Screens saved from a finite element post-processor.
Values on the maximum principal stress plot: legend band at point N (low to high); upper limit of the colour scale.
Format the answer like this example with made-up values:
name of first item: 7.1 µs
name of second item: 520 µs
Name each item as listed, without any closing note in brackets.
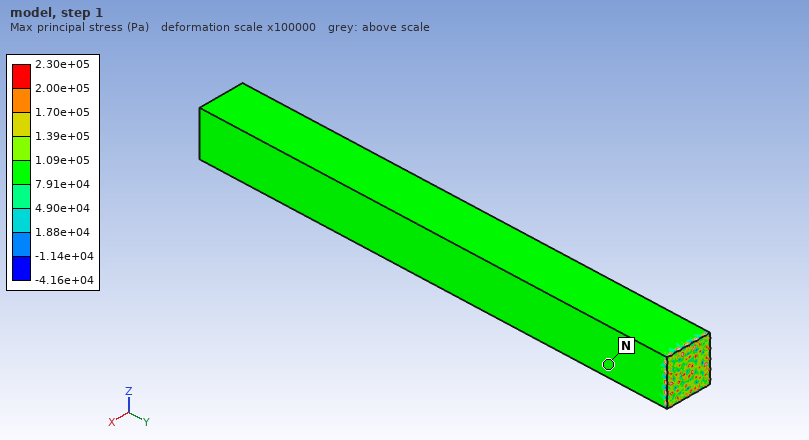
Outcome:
legend band at point N: 7.91e+04 to 1.09e+05 Pa
upper limit of the colour scale: 2.30e+05 Pa
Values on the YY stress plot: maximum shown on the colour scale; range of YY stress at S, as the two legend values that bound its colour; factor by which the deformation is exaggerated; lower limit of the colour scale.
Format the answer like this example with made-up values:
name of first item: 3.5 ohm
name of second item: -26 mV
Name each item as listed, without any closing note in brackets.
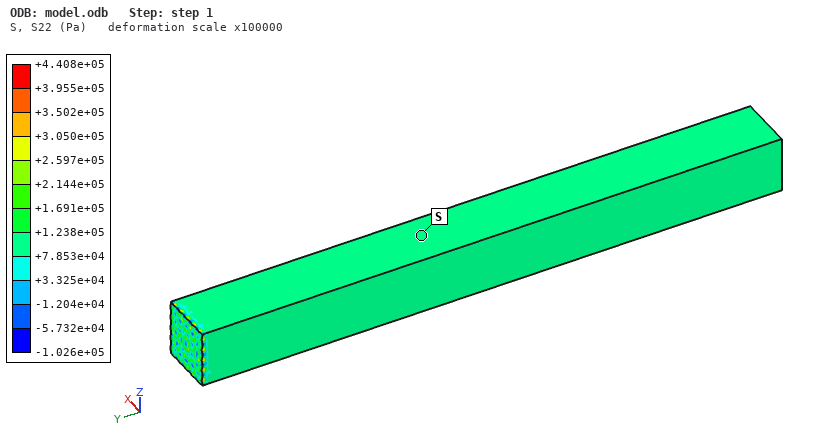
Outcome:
maximum shown on the colour scale: +4.408e+05 Pa
range of YY stress at S, as the two legend values that bound its colour: +7.853e+04 to +1.238e+05 Pa
factor by which the deformation is exaggerated: 100000
lower limit of the colour scale: -1.026e+05 Pa
